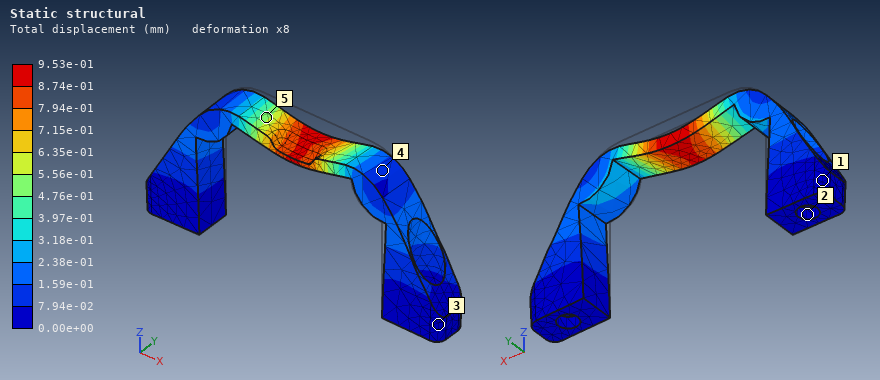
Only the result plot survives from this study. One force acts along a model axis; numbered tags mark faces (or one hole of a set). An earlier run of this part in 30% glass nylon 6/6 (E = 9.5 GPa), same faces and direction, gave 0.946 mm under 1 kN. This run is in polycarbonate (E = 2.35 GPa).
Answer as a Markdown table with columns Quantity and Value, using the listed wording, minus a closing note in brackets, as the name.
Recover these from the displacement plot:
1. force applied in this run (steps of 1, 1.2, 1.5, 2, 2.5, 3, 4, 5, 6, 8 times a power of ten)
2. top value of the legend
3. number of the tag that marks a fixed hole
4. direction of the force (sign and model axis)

| Quantity | Value |
|---|---|
| force applied in this run | 250 N |
| top value of the legend | 9.53e-01 mm |
| number of the tag that marks a fixed hole | 2 |
| direction of the force | -Z |
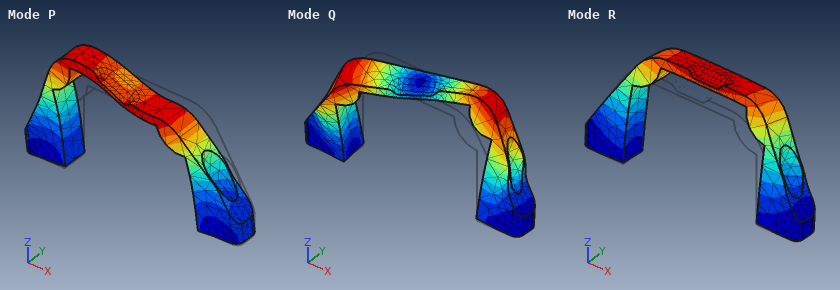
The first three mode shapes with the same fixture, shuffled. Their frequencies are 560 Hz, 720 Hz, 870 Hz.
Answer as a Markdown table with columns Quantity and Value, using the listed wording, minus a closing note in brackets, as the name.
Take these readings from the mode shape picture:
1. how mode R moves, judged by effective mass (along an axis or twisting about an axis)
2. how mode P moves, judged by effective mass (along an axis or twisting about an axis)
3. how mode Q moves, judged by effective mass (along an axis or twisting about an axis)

| Quantity | Value |
|---|---|
| how mode R moves, judged by effective mass | along Y |
| how mode P moves, judged by effective mass | along X |
| how mode Q moves, judged by effective mass | twisting about Z |
